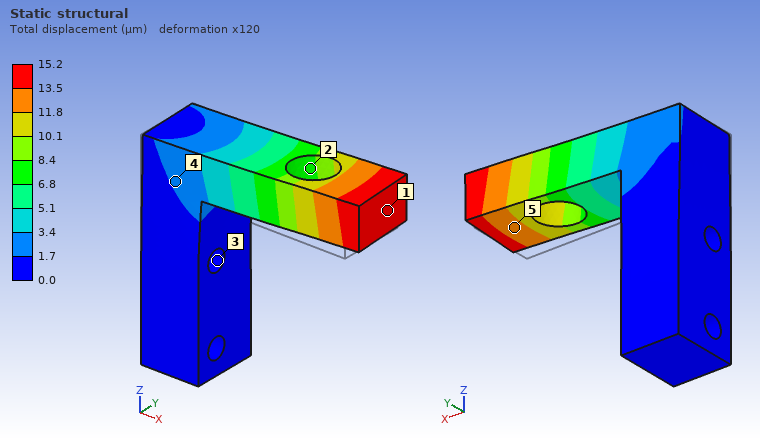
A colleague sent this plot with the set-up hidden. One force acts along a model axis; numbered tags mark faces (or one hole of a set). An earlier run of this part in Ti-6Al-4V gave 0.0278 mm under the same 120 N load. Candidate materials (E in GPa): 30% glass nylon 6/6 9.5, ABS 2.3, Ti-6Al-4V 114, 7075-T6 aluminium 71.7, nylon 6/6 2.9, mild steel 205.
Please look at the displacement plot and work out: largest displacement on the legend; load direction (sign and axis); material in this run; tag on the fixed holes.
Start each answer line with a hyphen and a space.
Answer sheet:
- 15.2 µm
- +Y
- mild steel
- 3
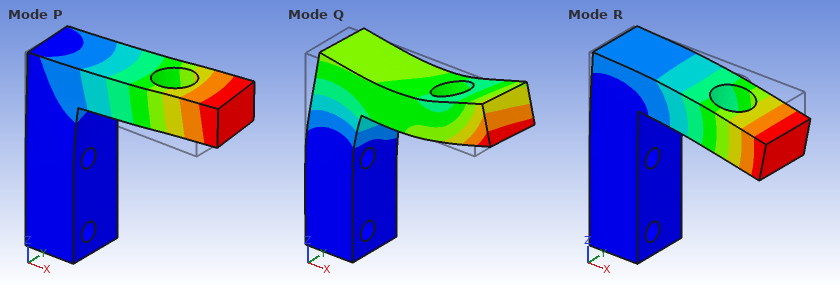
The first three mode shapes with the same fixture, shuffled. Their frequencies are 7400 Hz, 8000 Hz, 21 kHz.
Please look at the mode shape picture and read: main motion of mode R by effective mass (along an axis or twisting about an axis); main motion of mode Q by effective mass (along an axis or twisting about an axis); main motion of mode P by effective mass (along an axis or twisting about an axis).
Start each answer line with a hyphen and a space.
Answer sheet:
- along Z
- along X
- along Y
